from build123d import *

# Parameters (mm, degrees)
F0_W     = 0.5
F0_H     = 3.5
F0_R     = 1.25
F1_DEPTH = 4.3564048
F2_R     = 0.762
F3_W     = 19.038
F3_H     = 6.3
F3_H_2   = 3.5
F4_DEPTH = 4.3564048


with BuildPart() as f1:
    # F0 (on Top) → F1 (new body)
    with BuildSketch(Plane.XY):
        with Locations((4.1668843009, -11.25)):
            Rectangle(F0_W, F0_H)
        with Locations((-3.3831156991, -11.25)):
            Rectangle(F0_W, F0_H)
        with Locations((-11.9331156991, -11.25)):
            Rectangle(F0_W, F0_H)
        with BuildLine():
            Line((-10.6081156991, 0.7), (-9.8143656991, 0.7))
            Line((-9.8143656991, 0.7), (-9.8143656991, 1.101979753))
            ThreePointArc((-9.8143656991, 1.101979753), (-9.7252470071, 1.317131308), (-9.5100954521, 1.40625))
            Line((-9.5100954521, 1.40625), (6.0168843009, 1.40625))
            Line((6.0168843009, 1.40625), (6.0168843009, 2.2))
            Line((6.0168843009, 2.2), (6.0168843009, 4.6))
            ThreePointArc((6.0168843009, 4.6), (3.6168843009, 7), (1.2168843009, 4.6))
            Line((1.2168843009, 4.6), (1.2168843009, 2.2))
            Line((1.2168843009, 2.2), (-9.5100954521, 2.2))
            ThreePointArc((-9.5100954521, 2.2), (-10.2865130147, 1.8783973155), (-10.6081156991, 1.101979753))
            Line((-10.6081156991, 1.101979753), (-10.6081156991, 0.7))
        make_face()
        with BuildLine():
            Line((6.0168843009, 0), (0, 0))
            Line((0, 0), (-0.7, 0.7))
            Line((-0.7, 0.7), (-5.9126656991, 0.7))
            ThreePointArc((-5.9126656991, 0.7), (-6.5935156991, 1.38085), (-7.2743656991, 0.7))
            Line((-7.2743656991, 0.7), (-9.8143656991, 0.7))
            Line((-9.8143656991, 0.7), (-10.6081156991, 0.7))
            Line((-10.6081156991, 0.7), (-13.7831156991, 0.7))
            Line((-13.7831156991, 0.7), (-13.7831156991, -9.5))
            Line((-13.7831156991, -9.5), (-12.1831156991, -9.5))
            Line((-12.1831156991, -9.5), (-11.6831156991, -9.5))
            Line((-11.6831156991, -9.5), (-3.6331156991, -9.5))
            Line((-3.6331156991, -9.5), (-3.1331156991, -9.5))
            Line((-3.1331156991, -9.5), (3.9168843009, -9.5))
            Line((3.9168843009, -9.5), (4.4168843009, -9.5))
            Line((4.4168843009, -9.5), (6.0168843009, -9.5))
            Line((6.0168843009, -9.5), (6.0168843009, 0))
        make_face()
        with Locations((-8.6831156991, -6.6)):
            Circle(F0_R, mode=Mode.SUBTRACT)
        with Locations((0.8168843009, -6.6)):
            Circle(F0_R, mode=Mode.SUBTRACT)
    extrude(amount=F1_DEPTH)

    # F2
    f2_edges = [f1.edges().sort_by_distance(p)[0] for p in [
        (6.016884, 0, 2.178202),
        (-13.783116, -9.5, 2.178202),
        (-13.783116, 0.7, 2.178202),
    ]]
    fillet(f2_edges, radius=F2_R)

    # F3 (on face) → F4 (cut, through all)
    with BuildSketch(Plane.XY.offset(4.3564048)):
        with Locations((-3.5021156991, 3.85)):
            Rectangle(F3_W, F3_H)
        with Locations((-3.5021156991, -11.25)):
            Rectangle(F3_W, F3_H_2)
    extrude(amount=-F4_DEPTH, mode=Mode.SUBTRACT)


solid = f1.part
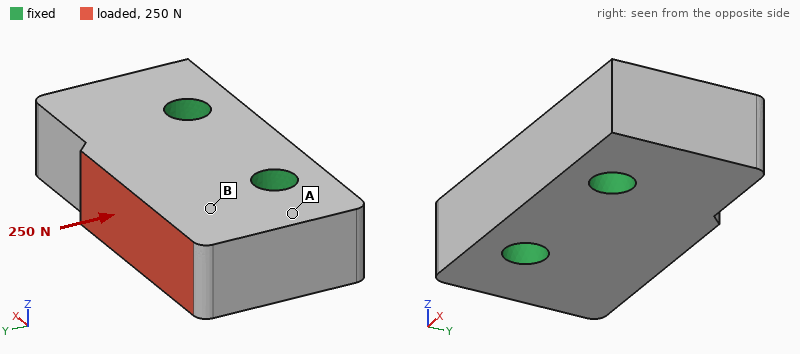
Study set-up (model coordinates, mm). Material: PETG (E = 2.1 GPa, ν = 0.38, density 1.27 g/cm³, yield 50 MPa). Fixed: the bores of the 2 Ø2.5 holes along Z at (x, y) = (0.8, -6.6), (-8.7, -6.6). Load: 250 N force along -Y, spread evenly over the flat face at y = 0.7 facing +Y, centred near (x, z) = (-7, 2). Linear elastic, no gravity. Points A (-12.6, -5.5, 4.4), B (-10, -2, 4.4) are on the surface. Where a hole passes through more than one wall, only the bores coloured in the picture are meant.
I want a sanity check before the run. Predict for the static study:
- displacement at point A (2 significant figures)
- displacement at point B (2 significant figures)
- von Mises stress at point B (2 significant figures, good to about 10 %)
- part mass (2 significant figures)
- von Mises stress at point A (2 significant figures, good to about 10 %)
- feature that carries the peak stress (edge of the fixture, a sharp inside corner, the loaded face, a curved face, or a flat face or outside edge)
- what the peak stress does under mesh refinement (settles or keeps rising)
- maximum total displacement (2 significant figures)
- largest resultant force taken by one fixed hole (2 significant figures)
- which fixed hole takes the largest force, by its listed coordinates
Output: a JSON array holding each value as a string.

["14 µm", "16 µm", "5.6 MPa", "1.0 g", "1.8 MPa", "edge of the fixture", "keeps rising", "25 µm", "190 N", "(-8.7, -6.6)"]
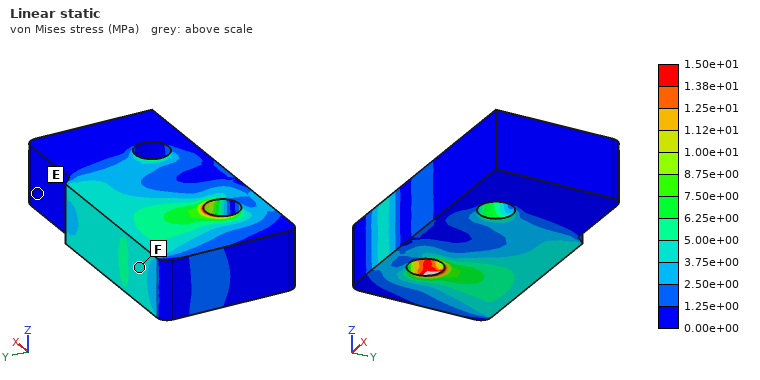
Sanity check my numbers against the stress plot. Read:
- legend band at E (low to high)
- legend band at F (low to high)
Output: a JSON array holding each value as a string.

["0.00e+00 to 1.25e+00 MPa", "3.75e+00 to 5.00e+00 MPa"]
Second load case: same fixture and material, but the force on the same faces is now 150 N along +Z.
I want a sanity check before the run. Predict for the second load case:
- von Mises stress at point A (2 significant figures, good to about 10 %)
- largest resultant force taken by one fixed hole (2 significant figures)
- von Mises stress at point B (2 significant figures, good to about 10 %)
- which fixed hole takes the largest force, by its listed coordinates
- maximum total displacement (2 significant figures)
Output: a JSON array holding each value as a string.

["9.0 MPa", "110 N", "9.3 MPa", "(-8.7, -6.6)", "0.13 mm"]
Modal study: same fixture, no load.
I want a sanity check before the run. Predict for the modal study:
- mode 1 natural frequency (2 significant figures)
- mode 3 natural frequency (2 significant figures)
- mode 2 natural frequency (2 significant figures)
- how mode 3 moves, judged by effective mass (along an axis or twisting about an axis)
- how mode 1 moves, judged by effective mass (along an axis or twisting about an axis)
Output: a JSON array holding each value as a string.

["14 kHz", "19 kHz", "16 kHz", "along X", "along Z"]
